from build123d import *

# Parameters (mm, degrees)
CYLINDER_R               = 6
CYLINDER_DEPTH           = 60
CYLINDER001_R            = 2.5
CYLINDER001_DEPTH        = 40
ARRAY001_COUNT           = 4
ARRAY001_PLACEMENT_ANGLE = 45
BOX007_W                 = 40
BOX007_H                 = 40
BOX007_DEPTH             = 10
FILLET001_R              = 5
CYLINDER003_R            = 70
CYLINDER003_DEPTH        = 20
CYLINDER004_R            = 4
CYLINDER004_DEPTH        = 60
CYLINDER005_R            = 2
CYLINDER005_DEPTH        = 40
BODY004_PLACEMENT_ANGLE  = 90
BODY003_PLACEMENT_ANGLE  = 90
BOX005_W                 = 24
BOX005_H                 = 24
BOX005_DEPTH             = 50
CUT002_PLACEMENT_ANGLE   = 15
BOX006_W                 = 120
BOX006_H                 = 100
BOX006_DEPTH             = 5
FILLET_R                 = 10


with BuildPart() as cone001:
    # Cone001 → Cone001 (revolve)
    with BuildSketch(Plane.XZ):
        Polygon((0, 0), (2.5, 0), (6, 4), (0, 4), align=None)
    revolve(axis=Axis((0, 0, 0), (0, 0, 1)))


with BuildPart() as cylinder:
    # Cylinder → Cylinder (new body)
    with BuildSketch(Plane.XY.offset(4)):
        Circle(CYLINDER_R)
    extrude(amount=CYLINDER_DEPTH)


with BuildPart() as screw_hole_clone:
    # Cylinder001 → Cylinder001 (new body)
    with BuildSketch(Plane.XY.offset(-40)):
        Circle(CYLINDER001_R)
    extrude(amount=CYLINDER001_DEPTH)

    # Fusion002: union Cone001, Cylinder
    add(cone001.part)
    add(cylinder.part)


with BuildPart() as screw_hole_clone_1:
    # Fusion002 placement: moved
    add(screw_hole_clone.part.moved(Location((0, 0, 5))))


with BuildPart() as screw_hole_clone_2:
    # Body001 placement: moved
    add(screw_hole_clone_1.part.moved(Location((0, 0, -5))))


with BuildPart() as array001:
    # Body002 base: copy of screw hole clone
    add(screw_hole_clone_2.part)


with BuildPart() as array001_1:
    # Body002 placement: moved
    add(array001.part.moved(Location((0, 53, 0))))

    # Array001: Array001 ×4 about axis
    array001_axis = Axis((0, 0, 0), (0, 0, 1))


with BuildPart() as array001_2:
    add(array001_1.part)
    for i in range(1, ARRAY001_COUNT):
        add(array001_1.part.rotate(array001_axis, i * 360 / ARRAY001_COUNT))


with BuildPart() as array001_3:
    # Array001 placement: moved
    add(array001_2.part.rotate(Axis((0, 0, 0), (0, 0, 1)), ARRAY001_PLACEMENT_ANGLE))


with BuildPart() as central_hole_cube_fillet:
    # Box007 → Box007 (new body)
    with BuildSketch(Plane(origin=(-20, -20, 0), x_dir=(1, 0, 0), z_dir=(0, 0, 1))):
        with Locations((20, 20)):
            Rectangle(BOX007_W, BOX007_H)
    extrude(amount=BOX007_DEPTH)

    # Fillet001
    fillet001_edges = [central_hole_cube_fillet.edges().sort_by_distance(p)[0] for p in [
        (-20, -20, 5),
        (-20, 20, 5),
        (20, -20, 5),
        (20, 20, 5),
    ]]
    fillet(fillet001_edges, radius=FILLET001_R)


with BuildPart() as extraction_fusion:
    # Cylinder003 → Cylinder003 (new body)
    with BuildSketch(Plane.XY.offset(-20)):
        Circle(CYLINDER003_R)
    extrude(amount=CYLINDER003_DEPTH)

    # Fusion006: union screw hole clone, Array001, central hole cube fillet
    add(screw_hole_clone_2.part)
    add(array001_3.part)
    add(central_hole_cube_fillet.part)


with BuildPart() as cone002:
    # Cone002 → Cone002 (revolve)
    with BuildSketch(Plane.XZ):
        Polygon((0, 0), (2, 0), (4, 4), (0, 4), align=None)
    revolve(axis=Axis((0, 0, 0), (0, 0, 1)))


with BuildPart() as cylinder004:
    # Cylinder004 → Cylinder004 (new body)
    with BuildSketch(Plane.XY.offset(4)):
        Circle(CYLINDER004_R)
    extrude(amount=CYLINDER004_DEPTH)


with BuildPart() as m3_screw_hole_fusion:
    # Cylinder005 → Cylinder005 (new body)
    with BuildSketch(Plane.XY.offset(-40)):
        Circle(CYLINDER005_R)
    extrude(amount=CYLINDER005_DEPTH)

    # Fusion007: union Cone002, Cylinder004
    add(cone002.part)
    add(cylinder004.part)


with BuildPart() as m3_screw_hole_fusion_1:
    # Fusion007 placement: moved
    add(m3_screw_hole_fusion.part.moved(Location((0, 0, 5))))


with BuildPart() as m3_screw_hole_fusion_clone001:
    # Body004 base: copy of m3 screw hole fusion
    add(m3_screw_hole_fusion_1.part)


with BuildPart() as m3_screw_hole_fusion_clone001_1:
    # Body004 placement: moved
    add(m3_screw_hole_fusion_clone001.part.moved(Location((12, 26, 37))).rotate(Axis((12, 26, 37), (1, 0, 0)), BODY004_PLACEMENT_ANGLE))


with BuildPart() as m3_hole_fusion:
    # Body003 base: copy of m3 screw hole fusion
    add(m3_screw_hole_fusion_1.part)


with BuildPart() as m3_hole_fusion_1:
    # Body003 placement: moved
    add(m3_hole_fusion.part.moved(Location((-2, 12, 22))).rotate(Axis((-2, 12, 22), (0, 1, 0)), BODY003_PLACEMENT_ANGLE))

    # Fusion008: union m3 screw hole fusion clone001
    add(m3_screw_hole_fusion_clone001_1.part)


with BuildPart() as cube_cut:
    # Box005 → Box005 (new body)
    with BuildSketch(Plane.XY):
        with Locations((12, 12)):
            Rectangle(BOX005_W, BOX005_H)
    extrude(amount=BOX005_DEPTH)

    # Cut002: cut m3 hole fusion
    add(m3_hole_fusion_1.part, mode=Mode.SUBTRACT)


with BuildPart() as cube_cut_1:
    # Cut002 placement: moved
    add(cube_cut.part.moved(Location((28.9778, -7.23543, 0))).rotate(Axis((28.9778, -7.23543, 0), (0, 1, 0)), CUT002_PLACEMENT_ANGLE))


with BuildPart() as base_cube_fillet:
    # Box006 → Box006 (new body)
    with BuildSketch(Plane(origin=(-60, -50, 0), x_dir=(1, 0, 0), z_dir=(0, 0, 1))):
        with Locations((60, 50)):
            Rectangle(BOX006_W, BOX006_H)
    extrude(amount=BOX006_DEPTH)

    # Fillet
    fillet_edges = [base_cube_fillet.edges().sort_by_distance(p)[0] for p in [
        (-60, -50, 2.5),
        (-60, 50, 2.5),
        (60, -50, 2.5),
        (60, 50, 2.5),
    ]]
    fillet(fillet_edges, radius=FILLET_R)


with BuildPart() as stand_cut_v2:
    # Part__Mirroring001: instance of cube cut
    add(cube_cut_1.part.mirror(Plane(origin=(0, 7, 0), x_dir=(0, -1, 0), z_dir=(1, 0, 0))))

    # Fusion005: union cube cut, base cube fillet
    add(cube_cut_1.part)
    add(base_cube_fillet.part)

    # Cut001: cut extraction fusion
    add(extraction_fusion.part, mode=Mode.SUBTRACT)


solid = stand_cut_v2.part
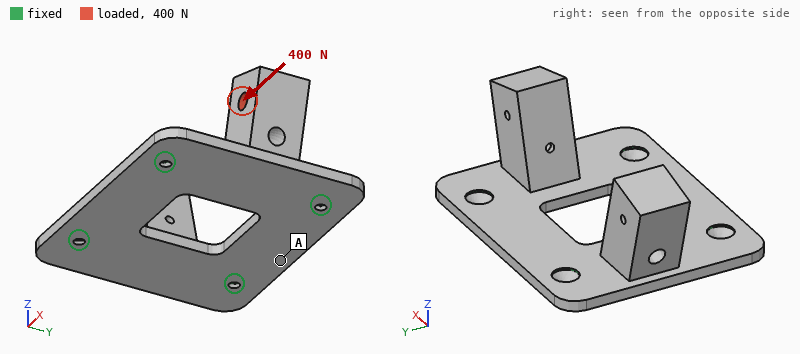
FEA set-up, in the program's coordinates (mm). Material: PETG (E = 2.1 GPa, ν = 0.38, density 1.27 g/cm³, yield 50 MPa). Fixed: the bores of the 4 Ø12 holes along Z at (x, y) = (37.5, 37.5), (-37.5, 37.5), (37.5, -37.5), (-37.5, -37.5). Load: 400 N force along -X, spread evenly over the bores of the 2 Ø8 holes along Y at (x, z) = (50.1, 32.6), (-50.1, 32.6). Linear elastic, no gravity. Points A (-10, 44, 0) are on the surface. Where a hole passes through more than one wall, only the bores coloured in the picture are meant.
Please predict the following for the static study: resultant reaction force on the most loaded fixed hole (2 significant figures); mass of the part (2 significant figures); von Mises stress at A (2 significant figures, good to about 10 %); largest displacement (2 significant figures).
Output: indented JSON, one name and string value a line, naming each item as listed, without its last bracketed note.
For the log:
{
  "resultant reaction force on the most loaded fixed hole": "120 N",
  "mass of the part": "120 g",
  "von Mises stress at A": "2.5 MPa",
  "largest displacement": "1.9 mm"
}
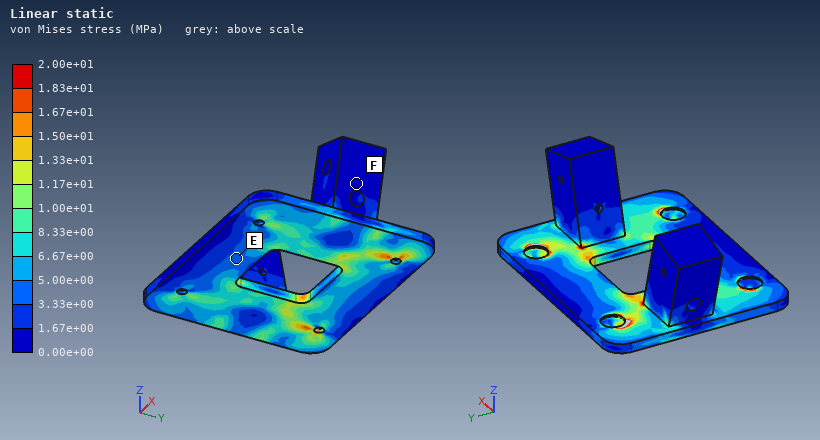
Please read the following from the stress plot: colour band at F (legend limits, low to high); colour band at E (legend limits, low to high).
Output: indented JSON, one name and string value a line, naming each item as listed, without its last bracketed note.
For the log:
{
  "colour band at F": "0.00e+00 to 1.67e+00 MPa",
  "colour band at E": "3.33e+00 to 5.00e+00 MPa"
}
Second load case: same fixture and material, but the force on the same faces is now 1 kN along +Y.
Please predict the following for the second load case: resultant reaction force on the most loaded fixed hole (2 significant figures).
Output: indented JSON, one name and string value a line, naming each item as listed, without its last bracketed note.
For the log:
{
  "resultant reaction force on the most loaded fixed hole": "430 N"
}
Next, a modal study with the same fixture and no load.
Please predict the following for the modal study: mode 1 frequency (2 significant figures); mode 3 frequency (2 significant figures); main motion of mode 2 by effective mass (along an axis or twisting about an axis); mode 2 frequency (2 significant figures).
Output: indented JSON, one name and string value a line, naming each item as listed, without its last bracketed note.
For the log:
{
  "mode 1 frequency": "360 Hz",
  "mode 3 frequency": "660 Hz",
  "main motion of mode 2 by effective mass": "along X",
  "mode 2 frequency": "390 Hz"
}
